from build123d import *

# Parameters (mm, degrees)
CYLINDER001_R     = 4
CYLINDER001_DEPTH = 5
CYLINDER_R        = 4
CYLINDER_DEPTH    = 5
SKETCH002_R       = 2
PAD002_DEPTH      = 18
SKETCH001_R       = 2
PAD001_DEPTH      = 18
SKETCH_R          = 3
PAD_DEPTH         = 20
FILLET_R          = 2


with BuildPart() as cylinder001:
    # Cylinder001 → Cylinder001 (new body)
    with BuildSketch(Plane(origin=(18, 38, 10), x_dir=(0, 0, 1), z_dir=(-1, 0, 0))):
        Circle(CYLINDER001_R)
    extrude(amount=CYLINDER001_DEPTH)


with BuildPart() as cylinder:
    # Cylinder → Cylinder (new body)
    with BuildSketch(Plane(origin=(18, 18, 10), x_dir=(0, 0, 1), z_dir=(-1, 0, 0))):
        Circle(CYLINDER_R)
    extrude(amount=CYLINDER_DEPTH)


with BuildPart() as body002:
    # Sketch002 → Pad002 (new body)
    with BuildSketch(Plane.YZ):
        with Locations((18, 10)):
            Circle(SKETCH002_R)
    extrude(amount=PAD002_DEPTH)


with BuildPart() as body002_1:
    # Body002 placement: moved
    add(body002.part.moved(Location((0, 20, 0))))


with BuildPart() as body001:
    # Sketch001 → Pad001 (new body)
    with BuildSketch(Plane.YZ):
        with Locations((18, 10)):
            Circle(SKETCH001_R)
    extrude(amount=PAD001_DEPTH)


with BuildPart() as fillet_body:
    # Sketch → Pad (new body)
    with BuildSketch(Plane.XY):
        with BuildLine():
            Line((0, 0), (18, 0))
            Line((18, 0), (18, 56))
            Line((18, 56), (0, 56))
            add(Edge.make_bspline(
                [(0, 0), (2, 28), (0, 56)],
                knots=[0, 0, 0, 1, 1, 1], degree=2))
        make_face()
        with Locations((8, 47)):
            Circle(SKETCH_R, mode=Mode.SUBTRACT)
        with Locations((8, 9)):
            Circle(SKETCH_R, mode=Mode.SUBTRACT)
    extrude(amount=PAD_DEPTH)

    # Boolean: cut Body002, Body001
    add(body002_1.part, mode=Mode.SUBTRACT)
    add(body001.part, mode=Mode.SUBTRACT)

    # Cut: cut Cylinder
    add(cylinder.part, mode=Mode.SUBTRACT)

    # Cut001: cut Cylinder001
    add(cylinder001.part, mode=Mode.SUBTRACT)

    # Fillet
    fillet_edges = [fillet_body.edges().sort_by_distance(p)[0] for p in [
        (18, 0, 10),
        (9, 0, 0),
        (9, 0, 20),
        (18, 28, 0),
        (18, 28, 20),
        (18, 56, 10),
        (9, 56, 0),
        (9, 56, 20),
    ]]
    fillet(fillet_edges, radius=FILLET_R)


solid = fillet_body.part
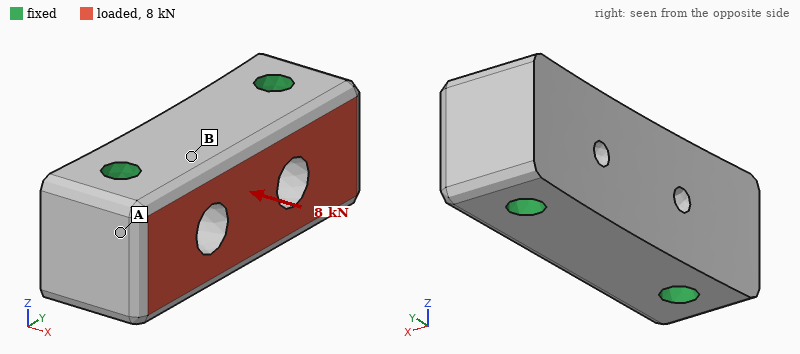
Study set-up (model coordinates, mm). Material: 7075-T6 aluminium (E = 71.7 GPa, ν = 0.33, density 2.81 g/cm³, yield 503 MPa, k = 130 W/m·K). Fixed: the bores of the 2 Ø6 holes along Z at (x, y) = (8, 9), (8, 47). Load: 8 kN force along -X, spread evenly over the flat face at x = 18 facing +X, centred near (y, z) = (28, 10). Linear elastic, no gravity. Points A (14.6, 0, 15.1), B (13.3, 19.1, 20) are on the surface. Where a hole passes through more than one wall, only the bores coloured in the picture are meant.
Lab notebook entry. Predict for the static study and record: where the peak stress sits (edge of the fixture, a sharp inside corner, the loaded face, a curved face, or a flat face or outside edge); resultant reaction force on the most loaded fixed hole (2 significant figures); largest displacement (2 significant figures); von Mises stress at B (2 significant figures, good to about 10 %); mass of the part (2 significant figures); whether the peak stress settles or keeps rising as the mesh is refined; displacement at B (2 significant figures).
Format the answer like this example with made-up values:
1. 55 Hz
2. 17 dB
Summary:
1. edge of the fixture
2. 4.0 kN
3. 5.9 µm
4. 10.0 MPa
5. 49 g
6. keeps rising
7. 3.9 µm
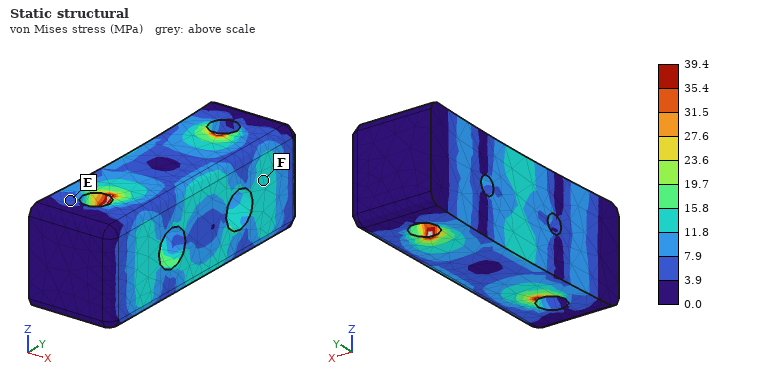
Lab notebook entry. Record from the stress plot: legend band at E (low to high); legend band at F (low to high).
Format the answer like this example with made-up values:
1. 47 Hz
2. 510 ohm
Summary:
1. 3.9 to 7.9 MPa
2. 11.8 to 15.8 MPa
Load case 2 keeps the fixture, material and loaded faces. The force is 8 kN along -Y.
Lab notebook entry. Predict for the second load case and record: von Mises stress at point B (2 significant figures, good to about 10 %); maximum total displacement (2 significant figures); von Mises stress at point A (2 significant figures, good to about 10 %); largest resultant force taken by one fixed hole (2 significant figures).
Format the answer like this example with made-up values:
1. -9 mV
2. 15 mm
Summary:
1. 14 MPa
2. 5.5 µm
3. 9.5 MPa
4. 4.3 kN
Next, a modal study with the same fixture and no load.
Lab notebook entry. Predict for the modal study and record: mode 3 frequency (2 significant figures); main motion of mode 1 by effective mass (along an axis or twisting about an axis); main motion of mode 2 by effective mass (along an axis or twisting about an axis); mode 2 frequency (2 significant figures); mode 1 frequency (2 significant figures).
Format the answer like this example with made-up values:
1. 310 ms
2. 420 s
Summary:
1. 38 kHz
2. along X
3. along Z
4. 32 kHz
5. 30 kHz
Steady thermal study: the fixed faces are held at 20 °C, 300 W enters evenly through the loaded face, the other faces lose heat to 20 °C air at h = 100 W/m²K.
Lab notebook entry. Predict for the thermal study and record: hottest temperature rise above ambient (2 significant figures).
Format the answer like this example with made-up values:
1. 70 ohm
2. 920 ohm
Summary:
1. 43 K
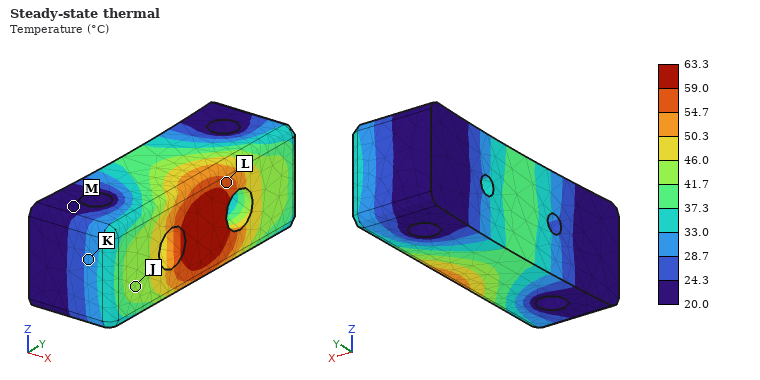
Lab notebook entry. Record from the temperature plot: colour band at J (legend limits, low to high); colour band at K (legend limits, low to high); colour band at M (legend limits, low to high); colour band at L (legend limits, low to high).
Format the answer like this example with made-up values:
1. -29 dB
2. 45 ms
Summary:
1. 41.7 to 46.0 °C
2. 28.7 to 33.0 °C
3. 20.0 to 24.3 °C
4. 54.7 to 59.0 °C
